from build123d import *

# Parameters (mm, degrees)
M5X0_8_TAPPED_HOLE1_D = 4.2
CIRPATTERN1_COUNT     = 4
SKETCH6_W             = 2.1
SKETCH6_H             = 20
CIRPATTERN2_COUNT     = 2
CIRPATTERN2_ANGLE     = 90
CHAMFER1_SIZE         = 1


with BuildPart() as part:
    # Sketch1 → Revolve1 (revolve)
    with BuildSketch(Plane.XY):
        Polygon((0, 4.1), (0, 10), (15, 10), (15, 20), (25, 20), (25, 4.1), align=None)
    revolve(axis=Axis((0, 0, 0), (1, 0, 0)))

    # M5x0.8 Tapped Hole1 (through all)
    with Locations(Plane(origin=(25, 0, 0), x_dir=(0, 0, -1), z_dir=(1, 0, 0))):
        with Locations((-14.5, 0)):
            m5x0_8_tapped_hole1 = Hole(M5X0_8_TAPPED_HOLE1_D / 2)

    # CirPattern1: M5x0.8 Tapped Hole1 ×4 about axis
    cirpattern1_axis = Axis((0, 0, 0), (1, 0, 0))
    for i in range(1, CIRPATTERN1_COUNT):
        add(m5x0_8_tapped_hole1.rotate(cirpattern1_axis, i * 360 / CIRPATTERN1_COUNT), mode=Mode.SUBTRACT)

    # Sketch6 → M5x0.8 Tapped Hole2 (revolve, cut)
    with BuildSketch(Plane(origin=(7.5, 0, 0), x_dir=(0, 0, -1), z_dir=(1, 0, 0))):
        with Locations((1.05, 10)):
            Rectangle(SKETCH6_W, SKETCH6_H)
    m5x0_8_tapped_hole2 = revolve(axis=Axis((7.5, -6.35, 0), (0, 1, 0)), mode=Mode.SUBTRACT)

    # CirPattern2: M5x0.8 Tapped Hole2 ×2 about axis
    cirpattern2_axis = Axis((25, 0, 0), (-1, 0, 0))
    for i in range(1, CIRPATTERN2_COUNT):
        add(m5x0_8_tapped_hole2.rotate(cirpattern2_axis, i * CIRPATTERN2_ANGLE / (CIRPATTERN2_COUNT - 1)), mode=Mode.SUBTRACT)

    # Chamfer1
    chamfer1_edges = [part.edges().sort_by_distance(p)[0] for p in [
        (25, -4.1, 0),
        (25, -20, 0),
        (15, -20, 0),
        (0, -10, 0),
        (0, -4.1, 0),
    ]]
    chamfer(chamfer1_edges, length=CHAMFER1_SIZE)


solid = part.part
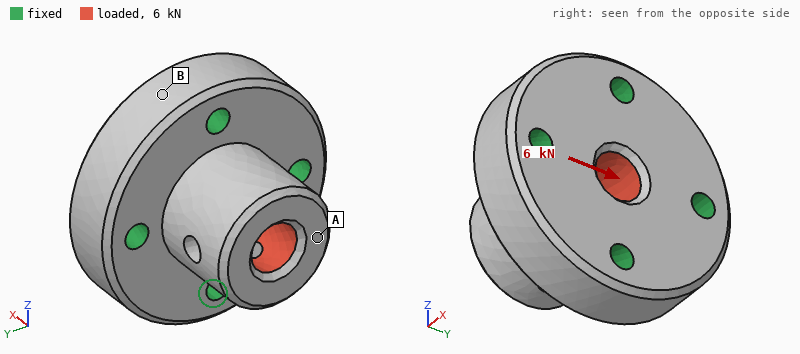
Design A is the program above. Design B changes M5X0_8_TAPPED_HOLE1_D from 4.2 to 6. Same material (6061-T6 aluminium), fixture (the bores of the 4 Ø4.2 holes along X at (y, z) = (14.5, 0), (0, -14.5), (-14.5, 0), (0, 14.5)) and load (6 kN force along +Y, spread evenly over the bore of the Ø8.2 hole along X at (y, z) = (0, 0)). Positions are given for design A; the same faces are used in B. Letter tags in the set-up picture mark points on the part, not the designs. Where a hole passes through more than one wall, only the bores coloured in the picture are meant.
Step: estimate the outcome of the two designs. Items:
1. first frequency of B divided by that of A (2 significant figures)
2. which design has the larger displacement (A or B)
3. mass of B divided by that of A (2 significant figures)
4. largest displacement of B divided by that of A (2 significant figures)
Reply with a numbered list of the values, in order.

1. 1.0
2. A
3. 0.96
4. 0.92
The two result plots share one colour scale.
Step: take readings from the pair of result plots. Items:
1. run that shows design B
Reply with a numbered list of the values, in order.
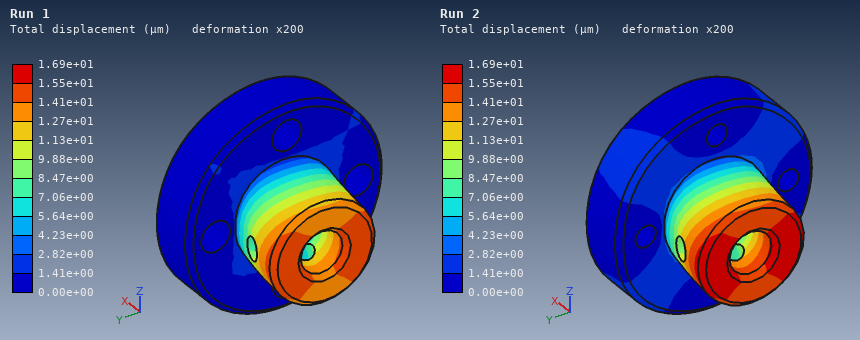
1. Run 1
